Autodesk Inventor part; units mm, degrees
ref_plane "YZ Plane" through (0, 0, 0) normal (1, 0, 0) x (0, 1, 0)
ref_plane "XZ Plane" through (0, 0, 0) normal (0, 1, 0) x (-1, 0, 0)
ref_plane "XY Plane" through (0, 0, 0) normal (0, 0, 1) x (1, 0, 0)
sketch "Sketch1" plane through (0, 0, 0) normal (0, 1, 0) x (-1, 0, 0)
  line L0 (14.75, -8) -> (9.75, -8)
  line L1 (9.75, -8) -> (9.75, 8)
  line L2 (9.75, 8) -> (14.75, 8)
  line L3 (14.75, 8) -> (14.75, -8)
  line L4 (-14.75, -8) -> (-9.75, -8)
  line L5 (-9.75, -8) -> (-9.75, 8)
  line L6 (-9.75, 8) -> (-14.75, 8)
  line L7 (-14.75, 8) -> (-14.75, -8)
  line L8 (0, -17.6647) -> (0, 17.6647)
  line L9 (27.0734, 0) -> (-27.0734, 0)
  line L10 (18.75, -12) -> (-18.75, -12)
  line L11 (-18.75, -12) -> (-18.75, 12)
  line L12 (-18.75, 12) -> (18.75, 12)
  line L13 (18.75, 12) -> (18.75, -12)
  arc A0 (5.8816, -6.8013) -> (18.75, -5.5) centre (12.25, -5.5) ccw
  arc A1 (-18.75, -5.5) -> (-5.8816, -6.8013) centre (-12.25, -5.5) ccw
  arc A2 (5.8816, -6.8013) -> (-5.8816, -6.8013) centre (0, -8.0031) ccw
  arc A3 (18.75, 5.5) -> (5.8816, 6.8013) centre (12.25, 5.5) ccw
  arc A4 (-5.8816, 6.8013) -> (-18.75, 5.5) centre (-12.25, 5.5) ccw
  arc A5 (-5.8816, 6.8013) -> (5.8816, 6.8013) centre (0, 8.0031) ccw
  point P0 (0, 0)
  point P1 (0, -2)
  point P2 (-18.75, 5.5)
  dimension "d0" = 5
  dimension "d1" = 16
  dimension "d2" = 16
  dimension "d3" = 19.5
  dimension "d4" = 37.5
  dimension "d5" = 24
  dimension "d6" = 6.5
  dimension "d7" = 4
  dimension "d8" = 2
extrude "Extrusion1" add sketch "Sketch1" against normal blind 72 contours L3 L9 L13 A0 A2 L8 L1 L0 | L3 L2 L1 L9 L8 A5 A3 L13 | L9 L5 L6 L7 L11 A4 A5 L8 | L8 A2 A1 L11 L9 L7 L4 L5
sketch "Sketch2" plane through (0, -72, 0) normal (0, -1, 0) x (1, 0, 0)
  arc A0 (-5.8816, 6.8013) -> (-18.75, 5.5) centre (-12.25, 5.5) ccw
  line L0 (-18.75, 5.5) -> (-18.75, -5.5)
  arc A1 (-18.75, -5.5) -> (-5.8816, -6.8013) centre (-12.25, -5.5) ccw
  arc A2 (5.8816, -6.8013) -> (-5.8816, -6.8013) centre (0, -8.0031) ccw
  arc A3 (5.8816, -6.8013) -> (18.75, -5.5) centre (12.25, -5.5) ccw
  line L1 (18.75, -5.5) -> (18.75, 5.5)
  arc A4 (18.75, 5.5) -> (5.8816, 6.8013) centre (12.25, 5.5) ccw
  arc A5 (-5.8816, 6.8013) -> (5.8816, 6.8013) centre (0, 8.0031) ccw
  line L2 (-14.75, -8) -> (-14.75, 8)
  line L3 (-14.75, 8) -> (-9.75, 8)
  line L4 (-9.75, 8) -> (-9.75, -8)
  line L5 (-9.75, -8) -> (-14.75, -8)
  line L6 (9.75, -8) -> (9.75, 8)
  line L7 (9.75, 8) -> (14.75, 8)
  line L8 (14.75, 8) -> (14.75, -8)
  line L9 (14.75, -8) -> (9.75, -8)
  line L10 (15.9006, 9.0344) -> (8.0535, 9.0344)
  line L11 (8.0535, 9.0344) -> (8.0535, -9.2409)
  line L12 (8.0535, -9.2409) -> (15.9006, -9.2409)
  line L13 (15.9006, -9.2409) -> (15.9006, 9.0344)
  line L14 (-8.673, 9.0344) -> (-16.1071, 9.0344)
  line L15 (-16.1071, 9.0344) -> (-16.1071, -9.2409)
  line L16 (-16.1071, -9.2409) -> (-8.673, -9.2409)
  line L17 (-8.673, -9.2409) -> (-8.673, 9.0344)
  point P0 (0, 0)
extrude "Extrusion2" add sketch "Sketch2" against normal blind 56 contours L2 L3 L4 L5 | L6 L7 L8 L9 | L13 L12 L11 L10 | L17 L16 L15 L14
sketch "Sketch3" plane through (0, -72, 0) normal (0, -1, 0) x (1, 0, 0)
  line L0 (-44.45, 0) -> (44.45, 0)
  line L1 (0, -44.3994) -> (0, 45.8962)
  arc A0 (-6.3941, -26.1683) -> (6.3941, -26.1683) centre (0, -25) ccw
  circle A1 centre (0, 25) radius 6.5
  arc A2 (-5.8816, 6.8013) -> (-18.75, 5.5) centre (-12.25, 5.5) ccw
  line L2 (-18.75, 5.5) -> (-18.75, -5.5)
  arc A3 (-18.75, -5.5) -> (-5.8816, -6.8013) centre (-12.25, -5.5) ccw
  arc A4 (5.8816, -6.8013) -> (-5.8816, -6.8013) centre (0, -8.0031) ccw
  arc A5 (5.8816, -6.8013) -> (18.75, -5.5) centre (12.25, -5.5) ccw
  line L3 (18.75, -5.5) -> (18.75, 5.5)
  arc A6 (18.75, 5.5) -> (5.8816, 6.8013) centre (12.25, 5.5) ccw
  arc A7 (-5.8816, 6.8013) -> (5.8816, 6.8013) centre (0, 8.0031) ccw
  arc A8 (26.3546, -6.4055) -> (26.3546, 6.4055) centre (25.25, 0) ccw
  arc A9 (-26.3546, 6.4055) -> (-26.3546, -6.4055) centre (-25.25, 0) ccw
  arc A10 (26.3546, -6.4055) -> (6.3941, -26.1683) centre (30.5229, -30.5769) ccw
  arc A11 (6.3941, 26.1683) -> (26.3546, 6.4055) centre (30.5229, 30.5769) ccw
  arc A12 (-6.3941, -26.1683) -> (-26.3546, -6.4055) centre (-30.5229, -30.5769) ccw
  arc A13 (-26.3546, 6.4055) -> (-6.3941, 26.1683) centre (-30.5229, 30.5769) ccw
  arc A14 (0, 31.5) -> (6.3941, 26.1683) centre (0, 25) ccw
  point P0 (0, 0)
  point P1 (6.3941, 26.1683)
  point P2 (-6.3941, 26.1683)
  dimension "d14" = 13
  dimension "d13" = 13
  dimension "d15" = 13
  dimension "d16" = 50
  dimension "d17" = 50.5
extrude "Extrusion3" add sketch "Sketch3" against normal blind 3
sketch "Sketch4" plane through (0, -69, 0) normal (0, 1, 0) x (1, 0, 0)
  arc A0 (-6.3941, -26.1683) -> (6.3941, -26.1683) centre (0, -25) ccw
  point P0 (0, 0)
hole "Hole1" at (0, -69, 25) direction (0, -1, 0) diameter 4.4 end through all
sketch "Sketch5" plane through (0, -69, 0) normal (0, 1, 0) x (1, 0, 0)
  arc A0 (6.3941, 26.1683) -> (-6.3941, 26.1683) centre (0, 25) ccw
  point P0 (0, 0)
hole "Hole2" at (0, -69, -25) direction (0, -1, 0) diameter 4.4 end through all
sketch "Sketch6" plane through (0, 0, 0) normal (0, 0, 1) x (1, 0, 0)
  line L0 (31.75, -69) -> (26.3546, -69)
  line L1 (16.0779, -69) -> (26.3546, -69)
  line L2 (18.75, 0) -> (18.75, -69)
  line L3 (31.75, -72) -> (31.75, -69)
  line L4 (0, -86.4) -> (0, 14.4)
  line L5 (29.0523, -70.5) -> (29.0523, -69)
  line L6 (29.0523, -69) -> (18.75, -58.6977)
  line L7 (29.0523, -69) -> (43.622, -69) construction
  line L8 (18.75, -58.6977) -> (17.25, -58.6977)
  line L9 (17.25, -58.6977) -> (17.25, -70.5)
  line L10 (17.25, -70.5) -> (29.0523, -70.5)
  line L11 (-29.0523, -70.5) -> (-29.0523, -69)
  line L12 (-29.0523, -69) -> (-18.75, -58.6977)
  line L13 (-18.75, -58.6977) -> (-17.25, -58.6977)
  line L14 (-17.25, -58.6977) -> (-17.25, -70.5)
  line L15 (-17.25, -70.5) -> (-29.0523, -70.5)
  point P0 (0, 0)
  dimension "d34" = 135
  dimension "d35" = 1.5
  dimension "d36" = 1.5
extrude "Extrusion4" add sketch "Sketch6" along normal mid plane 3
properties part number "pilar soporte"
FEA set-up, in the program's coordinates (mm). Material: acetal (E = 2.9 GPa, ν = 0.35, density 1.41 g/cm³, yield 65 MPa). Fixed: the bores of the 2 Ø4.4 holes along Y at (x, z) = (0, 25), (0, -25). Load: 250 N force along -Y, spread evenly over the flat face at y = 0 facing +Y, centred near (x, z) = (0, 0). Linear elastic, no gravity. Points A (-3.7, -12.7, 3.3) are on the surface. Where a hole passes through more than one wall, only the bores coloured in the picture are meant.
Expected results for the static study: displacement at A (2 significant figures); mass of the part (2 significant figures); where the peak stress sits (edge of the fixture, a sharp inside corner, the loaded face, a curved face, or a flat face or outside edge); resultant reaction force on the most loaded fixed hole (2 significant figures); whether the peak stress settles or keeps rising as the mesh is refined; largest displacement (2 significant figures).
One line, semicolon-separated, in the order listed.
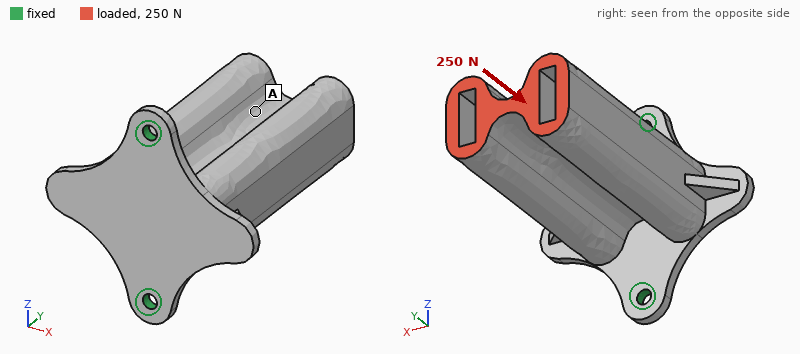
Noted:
0.39 mm; 65 g; edge of the fixture; 130 N; keeps rising; 0.39 mm
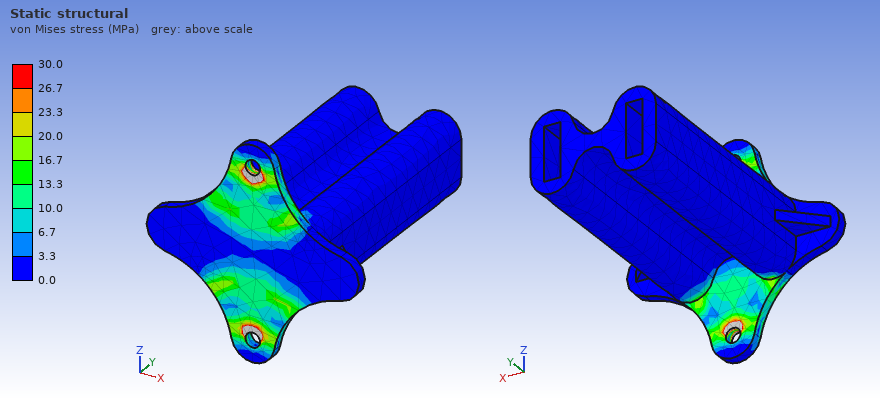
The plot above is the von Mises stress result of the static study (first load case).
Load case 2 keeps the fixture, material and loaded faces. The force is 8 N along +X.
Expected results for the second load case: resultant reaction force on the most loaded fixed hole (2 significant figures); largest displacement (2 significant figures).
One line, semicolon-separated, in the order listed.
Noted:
4.0 N; 1.2 mm
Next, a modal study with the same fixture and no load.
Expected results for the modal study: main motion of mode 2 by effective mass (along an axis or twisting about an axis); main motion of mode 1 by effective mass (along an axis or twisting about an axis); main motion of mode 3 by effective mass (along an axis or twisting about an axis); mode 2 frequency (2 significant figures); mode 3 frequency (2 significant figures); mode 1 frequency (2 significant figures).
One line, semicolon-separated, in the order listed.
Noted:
along Z; along X; along Y; 240 Hz; 510 Hz; 93 Hz
